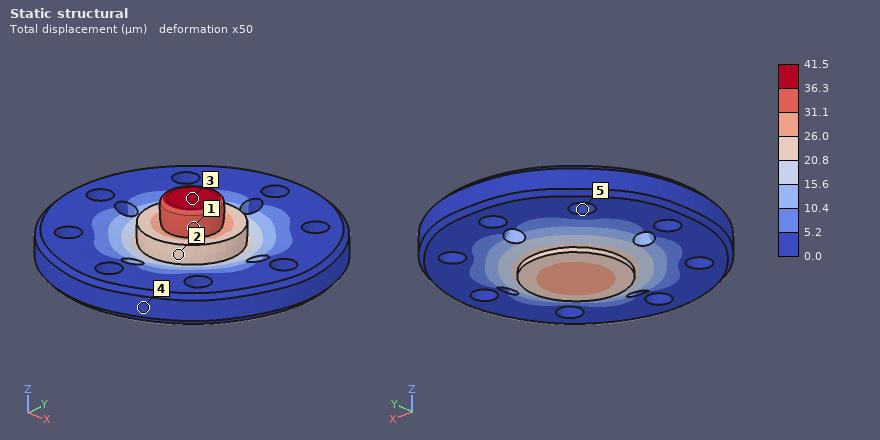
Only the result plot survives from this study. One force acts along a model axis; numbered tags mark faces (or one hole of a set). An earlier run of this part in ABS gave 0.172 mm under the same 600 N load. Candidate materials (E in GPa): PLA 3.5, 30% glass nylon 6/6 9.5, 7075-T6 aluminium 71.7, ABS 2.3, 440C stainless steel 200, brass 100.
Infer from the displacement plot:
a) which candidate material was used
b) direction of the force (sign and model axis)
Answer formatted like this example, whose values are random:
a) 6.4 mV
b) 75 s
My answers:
a) 30% glass nylon 6/6
b) -Z
